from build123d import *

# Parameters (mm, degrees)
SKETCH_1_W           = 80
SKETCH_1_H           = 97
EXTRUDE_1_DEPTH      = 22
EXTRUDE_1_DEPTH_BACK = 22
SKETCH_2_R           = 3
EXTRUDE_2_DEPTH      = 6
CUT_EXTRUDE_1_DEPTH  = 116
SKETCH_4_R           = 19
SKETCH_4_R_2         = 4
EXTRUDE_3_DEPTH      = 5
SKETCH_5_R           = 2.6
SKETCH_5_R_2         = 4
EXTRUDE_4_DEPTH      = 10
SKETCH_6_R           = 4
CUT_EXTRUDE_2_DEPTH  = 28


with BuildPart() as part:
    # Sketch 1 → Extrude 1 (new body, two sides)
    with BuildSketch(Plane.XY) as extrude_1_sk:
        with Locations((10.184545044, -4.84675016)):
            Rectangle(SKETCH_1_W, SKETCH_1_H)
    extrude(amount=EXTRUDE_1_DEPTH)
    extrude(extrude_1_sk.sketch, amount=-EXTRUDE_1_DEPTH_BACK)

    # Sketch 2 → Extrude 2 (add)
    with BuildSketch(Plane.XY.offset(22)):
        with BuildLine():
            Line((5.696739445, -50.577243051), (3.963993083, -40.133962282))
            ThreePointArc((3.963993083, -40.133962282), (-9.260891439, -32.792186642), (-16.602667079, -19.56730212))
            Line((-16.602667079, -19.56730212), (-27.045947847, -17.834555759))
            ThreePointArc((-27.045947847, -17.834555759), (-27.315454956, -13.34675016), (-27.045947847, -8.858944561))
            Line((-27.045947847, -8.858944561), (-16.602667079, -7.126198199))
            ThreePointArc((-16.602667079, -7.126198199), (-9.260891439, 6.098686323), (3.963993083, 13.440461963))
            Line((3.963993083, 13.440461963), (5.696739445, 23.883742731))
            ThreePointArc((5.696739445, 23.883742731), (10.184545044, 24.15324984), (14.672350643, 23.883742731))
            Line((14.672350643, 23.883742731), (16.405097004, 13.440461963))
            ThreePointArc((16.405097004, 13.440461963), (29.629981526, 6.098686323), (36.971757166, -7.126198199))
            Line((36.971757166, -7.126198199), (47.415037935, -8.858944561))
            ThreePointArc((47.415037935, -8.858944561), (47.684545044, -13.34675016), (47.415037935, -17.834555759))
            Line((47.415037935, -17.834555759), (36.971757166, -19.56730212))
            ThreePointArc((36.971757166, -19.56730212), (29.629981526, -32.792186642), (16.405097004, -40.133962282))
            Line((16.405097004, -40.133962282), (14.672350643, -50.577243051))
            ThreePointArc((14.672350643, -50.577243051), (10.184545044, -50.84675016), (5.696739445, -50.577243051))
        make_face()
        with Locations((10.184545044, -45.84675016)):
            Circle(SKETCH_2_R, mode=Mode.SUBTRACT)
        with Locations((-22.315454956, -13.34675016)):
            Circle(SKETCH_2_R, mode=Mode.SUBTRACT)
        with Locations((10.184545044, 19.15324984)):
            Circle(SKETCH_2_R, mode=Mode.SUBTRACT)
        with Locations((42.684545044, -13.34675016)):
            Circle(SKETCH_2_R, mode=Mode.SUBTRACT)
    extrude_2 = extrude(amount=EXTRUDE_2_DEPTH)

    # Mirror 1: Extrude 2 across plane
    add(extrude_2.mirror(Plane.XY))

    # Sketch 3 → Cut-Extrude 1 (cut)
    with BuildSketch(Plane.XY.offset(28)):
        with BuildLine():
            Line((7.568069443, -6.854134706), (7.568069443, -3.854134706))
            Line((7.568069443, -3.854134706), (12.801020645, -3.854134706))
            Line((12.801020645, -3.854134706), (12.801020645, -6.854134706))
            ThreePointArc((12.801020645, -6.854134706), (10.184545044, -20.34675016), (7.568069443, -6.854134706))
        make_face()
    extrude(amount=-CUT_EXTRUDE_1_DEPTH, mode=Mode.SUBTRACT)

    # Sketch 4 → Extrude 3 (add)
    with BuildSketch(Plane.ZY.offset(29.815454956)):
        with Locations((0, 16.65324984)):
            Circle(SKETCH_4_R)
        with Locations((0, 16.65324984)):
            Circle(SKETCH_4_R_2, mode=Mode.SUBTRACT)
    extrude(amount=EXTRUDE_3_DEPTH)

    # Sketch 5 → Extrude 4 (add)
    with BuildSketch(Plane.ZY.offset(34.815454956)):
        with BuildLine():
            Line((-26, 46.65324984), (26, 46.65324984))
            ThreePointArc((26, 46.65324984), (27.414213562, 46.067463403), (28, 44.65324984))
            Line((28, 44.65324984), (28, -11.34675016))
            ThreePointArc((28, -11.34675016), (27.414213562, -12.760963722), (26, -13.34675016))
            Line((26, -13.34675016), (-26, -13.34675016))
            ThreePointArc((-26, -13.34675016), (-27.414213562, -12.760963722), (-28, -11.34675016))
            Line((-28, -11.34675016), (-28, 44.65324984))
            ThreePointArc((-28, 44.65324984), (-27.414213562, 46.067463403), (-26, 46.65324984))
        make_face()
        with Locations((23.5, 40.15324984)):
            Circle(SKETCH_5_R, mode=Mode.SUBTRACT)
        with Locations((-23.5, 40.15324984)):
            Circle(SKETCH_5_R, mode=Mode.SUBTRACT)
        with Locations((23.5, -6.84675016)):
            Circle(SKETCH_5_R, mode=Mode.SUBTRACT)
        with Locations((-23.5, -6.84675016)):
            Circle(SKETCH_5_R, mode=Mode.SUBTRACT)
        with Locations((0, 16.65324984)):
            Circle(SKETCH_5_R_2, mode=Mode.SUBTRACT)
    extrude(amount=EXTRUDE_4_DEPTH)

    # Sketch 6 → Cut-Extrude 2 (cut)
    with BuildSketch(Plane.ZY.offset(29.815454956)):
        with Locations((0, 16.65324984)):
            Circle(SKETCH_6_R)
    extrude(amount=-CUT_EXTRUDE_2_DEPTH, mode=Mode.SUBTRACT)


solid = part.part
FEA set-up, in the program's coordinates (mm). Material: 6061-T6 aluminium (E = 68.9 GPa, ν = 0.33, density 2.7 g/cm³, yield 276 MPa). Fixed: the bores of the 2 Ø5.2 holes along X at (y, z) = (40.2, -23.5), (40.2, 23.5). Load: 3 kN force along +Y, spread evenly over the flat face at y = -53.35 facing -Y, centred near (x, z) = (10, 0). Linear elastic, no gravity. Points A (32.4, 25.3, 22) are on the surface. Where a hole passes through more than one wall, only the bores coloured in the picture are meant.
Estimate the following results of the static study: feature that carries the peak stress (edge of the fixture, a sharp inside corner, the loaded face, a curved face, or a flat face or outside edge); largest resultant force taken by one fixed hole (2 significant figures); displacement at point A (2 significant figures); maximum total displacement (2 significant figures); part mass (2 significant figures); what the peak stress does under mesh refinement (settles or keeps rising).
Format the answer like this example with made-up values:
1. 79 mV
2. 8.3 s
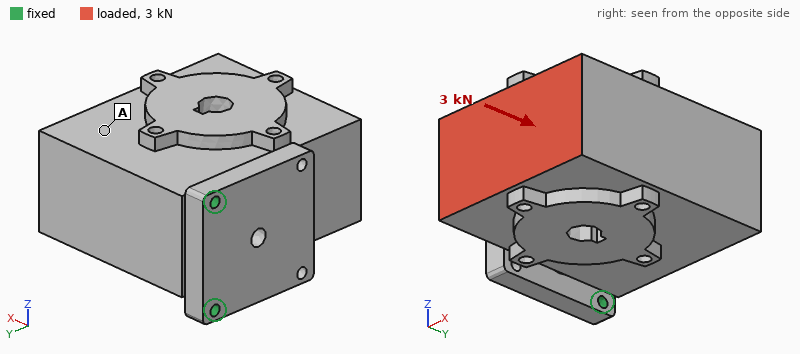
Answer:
1. edge of the fixture
2. 1.7 kN
3. 0.68 mm
4. 1.2 mm
5. 1.1 kg
6. keeps rising
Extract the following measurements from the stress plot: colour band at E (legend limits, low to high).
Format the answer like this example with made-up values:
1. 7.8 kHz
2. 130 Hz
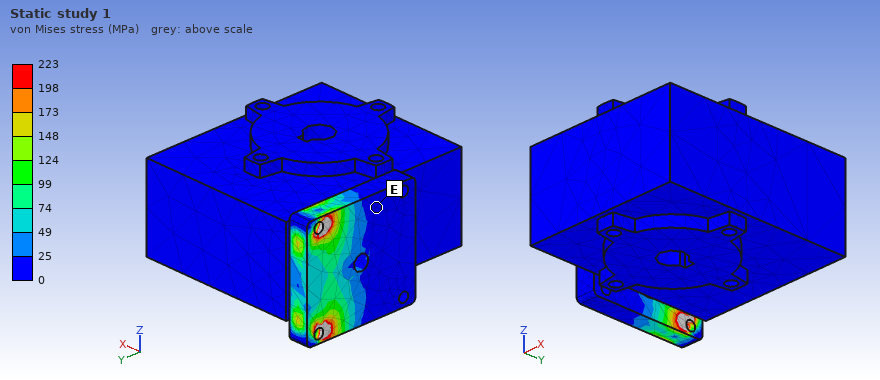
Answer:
1. 0 to 25 MPa
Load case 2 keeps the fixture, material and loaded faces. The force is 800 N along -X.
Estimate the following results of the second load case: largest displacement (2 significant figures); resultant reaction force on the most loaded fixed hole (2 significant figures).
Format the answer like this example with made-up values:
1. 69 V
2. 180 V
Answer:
1. 0.55 mm
2. 420 N
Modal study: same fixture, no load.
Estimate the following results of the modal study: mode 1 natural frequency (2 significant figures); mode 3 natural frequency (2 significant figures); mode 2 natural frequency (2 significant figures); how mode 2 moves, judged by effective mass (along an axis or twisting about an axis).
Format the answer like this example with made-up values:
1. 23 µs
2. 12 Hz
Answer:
1. 280 Hz
2. 2000 Hz
3. 750 Hz
4. along Z
